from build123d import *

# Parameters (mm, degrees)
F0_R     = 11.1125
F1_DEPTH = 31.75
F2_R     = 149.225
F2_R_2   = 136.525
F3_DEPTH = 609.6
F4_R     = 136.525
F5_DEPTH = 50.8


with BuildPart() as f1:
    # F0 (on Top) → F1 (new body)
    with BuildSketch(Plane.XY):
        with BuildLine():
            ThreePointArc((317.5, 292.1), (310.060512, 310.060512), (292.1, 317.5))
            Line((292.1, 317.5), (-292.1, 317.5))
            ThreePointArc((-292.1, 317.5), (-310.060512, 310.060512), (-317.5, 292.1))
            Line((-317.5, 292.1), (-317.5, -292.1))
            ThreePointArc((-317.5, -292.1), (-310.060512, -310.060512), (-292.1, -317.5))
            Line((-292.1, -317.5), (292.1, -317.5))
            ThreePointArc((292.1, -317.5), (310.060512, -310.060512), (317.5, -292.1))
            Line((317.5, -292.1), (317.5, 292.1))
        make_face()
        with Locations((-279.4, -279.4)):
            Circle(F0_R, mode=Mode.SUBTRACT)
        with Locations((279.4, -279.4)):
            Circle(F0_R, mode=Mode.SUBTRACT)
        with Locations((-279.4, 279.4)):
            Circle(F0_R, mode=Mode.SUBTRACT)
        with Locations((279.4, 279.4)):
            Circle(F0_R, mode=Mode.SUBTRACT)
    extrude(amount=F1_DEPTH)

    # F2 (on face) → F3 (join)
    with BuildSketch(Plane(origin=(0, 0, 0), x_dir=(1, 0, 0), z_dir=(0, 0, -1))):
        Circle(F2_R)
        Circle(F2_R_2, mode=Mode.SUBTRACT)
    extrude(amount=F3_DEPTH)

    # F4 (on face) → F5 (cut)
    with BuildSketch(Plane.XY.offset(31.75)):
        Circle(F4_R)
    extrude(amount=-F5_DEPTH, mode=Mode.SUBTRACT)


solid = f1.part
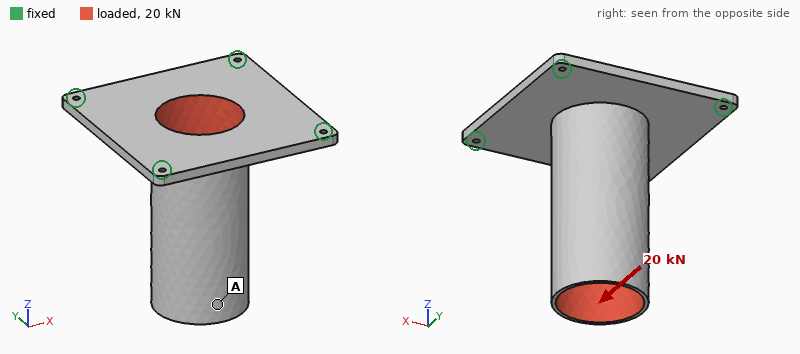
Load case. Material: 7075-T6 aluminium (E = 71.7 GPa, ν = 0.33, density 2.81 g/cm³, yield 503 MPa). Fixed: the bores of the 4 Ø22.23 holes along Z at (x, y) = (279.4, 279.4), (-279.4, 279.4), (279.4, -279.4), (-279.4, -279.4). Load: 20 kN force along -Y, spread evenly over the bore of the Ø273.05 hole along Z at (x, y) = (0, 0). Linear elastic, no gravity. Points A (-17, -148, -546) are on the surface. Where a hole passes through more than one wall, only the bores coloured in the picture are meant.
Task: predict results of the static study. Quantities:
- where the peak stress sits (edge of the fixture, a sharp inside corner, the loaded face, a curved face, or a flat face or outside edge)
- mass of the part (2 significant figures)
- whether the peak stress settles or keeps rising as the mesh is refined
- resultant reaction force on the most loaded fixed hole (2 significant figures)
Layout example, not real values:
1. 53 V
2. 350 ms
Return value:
1. edge of the fixture
2. 50 kg
3. keeps rising
4. 8.9 kN
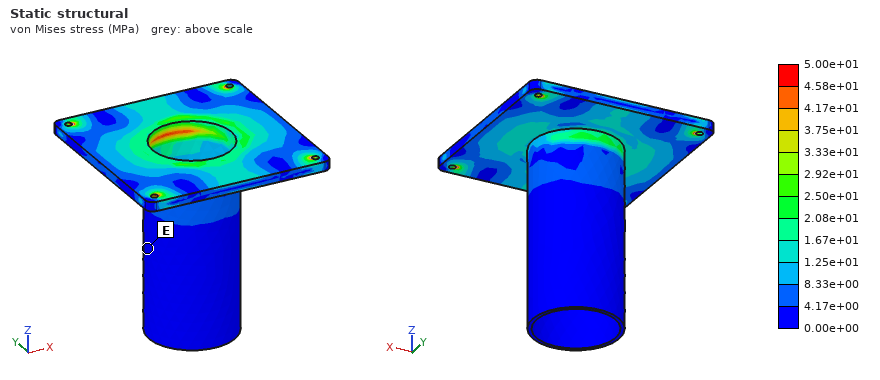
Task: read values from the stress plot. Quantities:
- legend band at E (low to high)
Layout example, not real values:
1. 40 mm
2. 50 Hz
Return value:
1. 0.00e+00 to 4.17e+00 MPa
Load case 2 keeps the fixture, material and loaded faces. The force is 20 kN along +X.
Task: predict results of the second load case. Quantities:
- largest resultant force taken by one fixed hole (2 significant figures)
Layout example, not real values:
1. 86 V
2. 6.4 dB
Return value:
1. 8.9 kN
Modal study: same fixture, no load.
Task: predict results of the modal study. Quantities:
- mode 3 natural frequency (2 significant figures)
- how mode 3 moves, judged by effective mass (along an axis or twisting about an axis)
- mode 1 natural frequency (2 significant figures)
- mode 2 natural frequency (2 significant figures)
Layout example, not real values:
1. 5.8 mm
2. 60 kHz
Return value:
1. 240 Hz
2. along Z
3. 160 Hz
4. 160 Hz
